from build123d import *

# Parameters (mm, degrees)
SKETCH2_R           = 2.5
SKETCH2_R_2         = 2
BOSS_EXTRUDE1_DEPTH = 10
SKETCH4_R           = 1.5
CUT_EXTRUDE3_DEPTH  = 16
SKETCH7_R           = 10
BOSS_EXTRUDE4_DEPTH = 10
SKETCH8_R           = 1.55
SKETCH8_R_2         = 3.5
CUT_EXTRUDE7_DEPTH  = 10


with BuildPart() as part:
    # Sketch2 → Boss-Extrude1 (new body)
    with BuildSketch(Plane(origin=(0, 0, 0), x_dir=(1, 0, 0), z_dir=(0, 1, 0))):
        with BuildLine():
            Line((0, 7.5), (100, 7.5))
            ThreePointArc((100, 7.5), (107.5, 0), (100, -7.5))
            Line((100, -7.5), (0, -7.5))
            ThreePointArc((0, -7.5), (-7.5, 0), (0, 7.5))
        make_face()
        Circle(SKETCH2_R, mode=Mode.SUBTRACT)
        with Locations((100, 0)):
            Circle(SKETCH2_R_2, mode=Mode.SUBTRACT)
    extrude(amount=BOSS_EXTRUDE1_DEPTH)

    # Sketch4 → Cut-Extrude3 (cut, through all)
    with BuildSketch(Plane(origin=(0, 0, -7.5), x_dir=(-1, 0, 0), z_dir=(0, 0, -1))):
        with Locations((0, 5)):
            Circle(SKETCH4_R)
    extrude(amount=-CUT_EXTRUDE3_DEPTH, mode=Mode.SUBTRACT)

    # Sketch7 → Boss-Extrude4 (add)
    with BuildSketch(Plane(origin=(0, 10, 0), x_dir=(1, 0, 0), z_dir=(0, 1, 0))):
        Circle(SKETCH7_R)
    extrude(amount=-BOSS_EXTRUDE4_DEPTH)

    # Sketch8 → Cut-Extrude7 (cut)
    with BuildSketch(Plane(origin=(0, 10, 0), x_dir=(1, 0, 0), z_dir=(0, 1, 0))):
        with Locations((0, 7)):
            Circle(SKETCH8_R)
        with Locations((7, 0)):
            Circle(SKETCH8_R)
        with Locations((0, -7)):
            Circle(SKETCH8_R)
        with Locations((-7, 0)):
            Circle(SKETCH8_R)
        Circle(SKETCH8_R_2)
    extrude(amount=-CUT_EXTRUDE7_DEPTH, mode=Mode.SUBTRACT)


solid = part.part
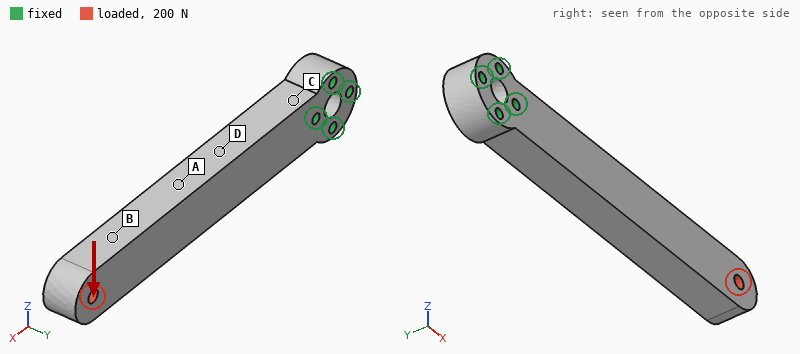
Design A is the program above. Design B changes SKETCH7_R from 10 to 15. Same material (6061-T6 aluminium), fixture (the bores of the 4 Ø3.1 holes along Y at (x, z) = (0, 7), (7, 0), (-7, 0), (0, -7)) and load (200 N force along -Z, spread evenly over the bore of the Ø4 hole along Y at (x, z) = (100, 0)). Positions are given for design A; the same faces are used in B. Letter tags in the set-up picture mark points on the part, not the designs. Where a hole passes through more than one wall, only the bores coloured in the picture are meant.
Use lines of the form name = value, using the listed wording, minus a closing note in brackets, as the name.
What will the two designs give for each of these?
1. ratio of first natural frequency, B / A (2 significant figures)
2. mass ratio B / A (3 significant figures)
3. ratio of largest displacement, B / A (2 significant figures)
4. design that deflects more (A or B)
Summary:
ratio of first natural frequency, B / A = 1.0
mass ratio B / A = 1.18
ratio of largest displacement, B / A = 0.88
design that deflects more = A
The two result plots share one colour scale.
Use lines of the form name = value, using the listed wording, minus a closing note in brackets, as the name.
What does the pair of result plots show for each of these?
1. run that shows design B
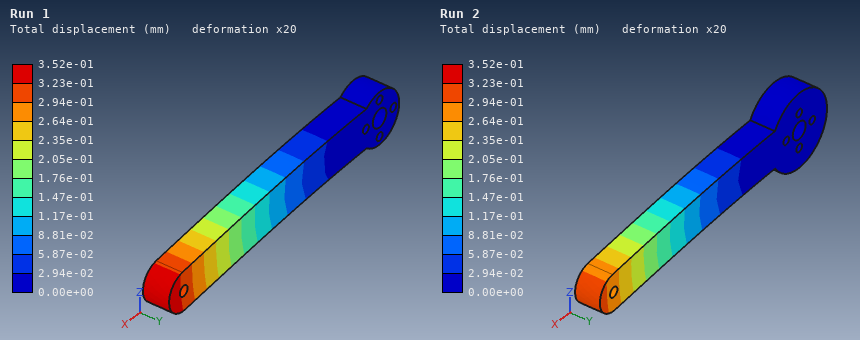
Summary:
run that shows design B = Run 2
